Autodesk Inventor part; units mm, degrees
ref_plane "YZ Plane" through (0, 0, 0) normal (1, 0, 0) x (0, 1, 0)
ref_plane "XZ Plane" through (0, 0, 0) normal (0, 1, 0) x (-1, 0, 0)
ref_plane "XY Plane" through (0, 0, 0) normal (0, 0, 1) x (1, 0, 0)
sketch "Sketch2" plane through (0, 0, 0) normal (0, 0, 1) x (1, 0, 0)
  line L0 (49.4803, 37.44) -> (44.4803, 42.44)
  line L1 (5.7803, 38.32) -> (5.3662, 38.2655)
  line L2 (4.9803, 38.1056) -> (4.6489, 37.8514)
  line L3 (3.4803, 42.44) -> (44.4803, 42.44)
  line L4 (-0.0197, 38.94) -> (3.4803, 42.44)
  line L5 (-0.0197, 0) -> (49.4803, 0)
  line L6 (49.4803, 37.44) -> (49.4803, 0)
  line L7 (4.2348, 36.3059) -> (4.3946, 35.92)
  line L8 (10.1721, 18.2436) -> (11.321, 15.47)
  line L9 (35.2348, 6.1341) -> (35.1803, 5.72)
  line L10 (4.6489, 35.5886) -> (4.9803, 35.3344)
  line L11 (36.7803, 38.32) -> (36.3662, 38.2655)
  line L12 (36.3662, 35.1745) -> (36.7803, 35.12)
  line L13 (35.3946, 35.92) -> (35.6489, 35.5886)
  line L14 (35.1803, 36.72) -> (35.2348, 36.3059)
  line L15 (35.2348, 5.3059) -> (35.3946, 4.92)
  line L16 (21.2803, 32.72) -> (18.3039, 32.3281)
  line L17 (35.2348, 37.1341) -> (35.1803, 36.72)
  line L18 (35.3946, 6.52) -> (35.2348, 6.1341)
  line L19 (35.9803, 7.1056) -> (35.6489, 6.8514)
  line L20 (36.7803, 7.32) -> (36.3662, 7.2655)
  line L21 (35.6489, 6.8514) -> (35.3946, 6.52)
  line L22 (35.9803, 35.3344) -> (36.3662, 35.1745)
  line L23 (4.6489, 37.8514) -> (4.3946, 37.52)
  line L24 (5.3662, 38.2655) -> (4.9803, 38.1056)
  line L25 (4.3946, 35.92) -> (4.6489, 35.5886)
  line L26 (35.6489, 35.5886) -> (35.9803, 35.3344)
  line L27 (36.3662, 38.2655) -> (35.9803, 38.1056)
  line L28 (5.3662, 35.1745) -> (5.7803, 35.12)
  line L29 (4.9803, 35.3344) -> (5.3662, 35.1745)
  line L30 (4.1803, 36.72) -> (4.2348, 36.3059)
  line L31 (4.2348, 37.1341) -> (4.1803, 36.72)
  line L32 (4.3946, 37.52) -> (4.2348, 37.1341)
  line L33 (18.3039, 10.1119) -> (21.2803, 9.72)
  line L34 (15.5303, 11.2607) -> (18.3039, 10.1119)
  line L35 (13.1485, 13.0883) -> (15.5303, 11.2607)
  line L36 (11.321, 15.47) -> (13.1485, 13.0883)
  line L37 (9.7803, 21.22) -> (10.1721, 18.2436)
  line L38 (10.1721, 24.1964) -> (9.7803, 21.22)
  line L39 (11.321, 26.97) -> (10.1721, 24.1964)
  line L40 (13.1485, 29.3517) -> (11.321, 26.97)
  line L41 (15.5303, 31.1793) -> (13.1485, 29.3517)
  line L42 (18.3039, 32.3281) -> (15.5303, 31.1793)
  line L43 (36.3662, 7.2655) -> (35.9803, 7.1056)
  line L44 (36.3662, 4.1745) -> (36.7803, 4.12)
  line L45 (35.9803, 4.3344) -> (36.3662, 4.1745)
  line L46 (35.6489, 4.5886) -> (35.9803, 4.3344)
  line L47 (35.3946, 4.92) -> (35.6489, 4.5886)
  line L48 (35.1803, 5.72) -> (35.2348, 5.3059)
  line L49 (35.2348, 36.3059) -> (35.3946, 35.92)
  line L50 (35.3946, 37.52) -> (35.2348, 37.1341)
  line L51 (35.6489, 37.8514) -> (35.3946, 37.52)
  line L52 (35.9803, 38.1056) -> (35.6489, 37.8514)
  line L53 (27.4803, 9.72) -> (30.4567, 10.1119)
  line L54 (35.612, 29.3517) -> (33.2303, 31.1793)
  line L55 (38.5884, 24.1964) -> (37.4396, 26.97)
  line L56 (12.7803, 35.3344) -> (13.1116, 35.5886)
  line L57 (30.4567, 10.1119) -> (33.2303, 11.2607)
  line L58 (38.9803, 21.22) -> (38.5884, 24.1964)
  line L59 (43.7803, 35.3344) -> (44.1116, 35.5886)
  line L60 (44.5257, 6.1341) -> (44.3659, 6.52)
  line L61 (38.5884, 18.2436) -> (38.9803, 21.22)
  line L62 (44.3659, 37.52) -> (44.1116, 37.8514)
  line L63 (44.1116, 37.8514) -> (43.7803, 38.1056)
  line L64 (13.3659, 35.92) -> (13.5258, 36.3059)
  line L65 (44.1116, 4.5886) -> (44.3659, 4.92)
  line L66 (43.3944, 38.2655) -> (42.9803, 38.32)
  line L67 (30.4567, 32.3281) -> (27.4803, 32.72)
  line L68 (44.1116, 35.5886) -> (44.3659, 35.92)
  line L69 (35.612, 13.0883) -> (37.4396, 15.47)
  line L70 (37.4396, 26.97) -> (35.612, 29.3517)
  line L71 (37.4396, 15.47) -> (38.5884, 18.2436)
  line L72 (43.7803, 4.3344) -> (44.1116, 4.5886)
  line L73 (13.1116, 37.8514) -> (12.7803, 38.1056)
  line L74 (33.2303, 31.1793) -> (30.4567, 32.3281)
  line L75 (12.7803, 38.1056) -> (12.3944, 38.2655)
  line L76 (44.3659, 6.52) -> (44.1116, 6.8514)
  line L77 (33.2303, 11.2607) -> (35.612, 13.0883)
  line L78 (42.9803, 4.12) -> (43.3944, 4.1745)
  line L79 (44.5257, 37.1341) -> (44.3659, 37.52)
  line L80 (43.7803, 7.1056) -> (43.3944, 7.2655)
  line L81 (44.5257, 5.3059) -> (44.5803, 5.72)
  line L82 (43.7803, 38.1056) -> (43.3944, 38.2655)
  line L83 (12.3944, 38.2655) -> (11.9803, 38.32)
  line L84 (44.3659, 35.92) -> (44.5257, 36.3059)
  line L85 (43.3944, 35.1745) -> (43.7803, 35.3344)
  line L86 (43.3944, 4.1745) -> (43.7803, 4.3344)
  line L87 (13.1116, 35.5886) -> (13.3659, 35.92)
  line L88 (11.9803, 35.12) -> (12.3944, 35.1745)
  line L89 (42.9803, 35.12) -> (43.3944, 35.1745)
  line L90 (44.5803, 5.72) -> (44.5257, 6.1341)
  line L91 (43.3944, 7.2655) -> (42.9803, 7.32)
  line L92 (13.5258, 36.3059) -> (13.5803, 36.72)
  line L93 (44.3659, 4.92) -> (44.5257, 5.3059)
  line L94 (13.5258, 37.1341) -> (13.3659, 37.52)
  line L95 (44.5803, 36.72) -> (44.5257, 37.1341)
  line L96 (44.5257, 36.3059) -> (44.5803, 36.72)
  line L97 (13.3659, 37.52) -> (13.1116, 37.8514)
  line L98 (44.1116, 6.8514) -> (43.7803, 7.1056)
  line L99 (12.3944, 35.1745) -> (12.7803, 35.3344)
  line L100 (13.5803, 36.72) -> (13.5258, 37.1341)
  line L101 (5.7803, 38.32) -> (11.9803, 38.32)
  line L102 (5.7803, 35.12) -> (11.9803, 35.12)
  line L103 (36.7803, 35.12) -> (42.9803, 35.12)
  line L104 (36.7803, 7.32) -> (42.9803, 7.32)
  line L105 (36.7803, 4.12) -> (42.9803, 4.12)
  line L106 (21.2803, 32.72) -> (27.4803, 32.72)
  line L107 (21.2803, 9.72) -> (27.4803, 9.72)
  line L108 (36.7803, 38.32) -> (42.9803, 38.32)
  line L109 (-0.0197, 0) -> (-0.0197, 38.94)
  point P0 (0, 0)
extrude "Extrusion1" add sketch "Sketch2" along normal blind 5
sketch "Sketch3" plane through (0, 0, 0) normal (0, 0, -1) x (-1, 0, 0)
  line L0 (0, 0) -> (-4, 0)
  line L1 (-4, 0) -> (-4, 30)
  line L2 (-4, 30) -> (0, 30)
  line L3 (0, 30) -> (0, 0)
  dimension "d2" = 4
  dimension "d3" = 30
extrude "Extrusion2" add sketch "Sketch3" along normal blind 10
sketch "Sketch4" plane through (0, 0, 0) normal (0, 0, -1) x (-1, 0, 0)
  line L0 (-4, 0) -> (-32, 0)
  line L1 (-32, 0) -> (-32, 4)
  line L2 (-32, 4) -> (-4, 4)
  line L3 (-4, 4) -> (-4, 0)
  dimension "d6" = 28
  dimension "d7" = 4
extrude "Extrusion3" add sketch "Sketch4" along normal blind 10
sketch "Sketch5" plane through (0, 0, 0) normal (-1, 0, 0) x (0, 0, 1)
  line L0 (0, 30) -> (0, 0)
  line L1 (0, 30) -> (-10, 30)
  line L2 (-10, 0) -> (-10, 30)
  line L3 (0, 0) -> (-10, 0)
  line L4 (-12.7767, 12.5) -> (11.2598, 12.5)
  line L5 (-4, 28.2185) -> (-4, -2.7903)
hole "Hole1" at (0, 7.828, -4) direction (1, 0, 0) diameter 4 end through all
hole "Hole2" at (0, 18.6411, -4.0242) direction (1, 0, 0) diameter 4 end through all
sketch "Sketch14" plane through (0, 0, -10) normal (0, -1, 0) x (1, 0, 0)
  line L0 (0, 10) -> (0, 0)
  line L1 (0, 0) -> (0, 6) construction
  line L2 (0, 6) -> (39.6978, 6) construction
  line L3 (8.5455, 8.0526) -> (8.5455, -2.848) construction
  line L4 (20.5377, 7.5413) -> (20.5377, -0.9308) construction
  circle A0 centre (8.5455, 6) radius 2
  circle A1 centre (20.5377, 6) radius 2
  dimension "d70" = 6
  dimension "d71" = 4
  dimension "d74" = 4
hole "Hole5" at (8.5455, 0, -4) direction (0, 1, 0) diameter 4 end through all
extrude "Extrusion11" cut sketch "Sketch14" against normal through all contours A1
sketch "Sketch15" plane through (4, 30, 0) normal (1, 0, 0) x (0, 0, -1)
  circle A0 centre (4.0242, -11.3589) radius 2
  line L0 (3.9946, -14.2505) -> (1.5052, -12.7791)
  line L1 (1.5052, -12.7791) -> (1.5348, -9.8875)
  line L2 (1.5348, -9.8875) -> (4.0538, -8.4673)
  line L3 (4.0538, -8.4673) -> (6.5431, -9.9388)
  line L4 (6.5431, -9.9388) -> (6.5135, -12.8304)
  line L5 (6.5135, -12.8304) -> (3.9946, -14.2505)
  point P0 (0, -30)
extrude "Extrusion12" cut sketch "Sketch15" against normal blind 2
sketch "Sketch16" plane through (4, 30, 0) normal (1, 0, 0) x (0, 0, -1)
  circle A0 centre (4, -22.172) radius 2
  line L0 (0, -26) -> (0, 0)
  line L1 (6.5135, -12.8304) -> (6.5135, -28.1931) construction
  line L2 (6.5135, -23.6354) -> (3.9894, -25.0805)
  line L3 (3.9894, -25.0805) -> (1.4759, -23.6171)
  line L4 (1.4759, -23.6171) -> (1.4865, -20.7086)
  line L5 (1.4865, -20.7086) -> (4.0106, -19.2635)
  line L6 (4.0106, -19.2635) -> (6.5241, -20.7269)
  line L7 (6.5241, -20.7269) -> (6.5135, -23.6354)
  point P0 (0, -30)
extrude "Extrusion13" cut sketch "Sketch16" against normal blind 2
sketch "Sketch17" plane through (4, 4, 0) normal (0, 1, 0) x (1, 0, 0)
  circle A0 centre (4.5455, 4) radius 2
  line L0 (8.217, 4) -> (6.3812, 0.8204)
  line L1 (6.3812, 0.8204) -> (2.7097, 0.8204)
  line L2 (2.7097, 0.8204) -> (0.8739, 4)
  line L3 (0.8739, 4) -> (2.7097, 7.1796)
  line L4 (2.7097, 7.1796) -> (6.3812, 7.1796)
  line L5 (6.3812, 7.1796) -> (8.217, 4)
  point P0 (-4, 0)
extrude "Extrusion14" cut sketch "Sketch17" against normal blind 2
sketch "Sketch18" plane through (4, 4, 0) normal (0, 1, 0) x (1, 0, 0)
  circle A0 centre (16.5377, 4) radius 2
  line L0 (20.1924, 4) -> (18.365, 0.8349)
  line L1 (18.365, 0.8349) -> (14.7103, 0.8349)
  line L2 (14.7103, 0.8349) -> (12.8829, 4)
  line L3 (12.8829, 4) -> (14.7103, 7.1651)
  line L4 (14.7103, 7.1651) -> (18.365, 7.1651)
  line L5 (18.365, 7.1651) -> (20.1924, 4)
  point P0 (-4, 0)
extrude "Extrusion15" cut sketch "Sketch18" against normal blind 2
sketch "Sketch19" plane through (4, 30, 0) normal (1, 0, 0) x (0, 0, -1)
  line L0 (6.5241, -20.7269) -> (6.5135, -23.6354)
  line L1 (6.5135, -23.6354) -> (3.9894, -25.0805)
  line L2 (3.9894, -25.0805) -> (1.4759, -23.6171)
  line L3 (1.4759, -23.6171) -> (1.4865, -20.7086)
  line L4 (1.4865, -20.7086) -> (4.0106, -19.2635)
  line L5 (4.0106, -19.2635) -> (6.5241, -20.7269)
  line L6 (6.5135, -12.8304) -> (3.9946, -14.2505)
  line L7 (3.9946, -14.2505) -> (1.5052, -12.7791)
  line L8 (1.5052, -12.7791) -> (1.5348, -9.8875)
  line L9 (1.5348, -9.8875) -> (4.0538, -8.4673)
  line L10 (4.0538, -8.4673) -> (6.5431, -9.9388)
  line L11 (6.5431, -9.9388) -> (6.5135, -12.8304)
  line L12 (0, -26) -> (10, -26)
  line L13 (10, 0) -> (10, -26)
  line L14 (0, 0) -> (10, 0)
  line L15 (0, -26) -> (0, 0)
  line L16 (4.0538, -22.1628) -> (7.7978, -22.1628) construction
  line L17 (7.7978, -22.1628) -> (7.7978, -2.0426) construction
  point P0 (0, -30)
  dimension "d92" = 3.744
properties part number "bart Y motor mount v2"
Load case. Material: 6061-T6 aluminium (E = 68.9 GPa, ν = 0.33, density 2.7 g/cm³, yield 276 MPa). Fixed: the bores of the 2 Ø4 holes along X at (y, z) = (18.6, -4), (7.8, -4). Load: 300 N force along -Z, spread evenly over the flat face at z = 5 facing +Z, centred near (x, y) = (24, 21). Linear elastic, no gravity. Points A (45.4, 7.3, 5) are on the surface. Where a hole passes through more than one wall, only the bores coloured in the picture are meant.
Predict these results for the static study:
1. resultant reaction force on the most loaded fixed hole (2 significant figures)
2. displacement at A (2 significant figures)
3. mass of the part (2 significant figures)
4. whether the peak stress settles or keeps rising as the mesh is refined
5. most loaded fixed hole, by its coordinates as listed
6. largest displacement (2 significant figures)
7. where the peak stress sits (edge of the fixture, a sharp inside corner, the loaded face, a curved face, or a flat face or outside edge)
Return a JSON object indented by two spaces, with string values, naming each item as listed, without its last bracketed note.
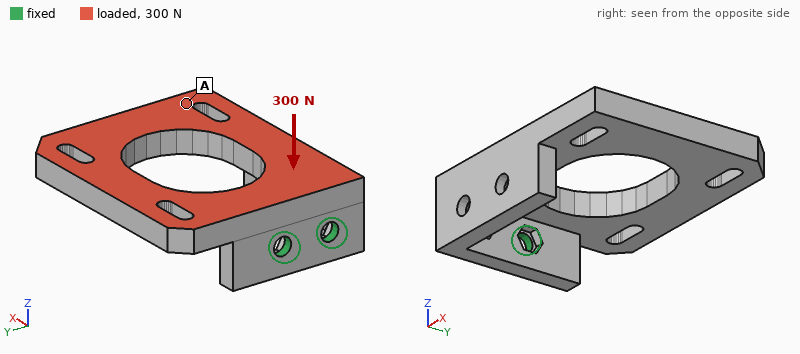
{
  "resultant reaction force on the most loaded fixed hole": "360 N",
  "displacement at A": "0.25 mm",
  "mass of the part": "25 g",
  "whether the peak stress settles or keeps rising as the mesh is refined": "keeps rising",
  "most loaded fixed hole, by its coordinates as listed": "(18.6, -4)",
  "largest displacement": "0.38 mm",
  "where the peak stress sits": "edge of the fixture"
}
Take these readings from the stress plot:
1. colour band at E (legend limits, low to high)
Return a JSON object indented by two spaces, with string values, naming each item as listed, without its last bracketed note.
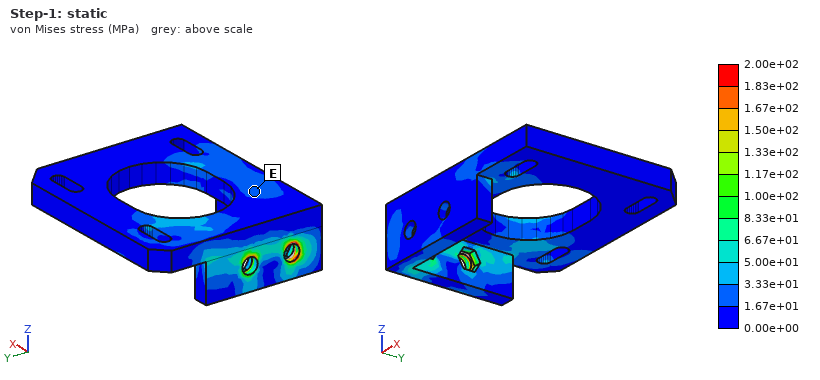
{
  "colour band at E": "1.67e+01 to 3.33e+01 MPa"
}
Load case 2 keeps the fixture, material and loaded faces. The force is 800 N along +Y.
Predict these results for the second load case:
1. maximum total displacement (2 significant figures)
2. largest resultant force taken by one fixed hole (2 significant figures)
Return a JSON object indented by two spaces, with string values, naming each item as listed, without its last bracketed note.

{
  "maximum total displacement": "0.20 mm",
  "largest resultant force taken by one fixed hole": "1.5 kN"
}
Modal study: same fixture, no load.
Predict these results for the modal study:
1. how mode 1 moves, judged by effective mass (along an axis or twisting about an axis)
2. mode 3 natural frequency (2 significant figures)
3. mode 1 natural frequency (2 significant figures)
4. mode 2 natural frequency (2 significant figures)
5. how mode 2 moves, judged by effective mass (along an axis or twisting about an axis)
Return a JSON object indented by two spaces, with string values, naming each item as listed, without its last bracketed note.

{
  "how mode 1 moves, judged by effective mass": "along Z",
  "mode 3 natural frequency": "3600 Hz",
  "mode 1 natural frequency": "1300 Hz",
  "mode 2 natural frequency": "2300 Hz",
  "how mode 2 moves, judged by effective mass": "along Y"
}
